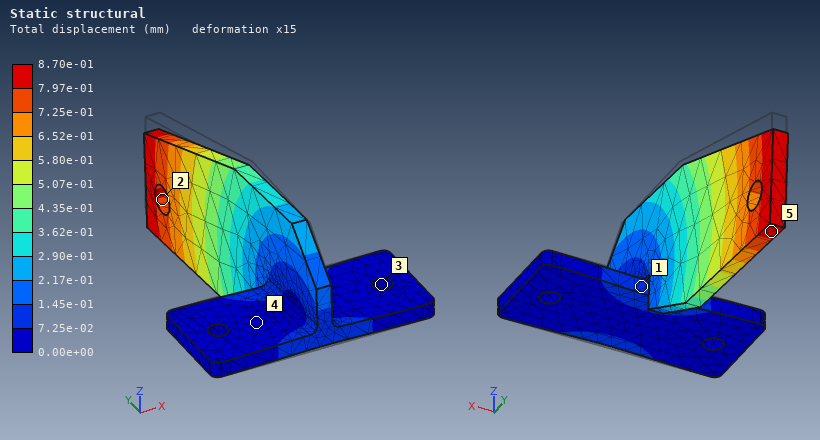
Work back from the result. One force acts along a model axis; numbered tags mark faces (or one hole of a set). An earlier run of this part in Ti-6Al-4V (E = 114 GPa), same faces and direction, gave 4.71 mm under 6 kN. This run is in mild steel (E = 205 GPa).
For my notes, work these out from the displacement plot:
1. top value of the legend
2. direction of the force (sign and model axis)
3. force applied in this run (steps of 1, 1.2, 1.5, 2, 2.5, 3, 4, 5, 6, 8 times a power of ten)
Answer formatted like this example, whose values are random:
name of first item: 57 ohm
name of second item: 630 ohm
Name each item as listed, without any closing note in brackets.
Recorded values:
top value of the legend: 8.70e-01 mm
direction of the force: -Z
force applied in this run: 2 kN
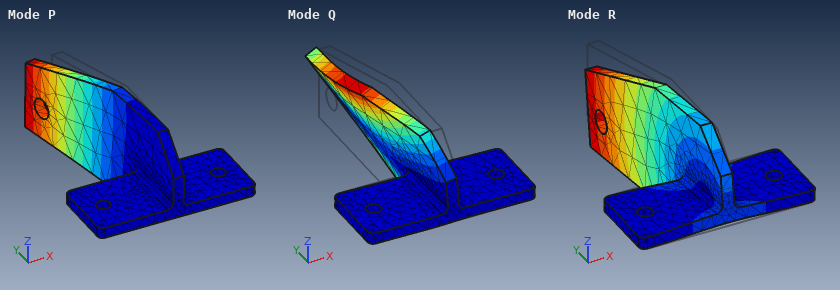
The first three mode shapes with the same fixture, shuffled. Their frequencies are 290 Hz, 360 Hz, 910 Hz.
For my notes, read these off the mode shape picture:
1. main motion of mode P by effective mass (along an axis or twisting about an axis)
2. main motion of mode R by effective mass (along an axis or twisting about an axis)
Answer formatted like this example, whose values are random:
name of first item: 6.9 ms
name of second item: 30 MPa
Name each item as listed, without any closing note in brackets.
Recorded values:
main motion of mode P by effective mass: along X
main motion of mode R by effective mass: along Z
